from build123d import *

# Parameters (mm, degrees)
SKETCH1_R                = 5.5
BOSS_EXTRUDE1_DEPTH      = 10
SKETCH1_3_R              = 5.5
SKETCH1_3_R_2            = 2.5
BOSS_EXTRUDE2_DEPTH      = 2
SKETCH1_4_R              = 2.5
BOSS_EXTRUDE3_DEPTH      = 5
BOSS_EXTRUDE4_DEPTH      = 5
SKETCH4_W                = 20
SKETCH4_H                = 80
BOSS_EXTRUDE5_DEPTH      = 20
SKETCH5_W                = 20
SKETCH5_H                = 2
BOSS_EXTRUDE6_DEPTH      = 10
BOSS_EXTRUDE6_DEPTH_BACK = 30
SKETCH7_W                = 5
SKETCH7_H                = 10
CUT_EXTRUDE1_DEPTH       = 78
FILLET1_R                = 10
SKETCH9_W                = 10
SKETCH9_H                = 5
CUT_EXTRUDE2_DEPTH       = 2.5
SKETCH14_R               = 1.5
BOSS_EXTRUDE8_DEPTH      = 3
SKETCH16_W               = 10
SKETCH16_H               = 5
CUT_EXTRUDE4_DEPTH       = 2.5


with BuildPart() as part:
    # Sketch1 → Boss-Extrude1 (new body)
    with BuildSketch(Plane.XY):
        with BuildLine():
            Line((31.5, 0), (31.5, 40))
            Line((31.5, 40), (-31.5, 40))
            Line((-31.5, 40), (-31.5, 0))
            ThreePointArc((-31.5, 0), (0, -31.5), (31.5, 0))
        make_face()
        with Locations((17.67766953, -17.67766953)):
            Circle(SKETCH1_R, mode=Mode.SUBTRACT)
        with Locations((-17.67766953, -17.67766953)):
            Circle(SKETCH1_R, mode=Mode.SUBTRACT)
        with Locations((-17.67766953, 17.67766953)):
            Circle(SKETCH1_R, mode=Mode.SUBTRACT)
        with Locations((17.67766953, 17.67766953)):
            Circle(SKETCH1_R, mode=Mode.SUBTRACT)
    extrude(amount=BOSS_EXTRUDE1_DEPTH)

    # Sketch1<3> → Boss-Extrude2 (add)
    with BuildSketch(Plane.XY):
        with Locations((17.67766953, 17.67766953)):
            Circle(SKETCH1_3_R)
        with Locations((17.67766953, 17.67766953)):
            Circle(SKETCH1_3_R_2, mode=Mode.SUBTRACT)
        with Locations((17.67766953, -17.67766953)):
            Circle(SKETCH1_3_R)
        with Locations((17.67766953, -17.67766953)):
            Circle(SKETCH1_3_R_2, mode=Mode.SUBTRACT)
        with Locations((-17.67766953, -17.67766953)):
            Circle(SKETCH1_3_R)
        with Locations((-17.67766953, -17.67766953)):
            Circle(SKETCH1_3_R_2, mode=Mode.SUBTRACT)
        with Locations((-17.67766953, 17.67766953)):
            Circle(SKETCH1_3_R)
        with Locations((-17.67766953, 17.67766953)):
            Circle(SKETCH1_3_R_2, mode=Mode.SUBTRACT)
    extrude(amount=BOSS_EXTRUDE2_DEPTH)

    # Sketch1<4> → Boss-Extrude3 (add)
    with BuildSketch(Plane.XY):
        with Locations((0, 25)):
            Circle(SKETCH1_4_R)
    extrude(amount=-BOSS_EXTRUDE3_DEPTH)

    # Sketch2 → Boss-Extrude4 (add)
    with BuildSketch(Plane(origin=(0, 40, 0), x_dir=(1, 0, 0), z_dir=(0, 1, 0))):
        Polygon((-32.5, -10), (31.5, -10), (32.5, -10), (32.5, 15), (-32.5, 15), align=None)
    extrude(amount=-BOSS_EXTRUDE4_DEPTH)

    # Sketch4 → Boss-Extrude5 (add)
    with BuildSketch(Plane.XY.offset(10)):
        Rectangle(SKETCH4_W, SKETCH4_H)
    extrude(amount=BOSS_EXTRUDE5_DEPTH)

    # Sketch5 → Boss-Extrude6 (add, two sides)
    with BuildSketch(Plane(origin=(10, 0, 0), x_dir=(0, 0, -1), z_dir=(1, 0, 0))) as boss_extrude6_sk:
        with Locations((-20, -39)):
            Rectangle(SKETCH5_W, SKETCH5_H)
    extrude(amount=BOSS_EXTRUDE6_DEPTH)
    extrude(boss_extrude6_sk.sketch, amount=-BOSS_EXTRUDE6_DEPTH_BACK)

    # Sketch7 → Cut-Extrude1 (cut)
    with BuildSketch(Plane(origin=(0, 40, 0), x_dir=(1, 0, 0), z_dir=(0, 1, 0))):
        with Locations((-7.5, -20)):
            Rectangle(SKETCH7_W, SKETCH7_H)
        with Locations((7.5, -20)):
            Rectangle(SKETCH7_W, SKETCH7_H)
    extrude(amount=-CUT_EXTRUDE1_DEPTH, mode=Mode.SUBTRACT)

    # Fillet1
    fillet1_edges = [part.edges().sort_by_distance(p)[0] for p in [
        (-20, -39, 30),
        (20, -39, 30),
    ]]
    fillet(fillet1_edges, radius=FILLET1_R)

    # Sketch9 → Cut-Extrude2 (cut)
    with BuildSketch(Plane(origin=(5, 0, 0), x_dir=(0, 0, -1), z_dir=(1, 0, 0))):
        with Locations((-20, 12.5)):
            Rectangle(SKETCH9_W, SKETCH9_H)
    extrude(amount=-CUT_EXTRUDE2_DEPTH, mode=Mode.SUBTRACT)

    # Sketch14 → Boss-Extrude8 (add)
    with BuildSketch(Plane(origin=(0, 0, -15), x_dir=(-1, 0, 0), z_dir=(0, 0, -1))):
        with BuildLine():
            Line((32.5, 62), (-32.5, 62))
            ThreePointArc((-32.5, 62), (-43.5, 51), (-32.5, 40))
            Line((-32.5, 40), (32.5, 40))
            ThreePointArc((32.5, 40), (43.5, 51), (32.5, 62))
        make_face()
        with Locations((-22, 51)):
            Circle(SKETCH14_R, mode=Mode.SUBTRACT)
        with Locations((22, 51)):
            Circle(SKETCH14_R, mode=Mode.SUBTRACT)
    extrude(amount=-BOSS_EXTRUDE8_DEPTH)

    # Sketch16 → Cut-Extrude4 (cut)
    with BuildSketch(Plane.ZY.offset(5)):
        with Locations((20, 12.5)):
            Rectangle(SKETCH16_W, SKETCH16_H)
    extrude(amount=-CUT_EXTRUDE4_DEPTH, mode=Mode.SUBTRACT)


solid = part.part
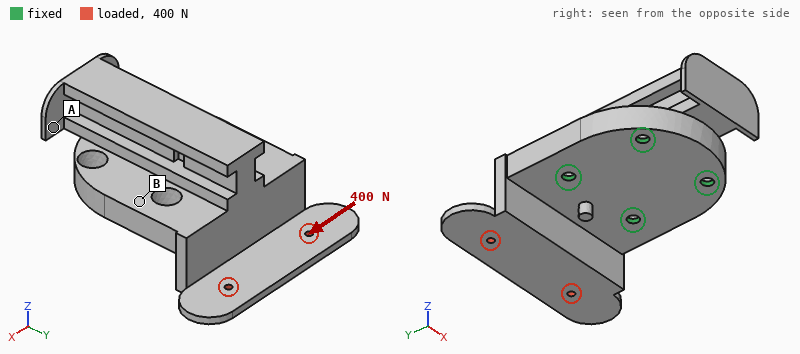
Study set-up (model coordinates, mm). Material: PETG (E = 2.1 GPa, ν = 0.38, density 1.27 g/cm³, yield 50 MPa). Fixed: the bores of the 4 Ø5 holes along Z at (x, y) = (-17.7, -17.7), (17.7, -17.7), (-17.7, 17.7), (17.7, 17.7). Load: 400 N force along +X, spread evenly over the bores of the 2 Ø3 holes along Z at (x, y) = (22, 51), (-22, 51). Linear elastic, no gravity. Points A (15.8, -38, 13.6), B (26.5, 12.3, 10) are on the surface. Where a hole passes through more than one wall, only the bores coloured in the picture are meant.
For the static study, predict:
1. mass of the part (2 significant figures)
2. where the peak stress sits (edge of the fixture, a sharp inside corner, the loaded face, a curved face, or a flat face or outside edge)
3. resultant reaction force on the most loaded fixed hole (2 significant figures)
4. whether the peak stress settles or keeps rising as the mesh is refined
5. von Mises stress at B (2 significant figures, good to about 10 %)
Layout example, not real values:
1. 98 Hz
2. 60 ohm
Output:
1. 92 g
2. edge of the fixture
3. 340 N
4. keeps rising
5. 3.2 MPa
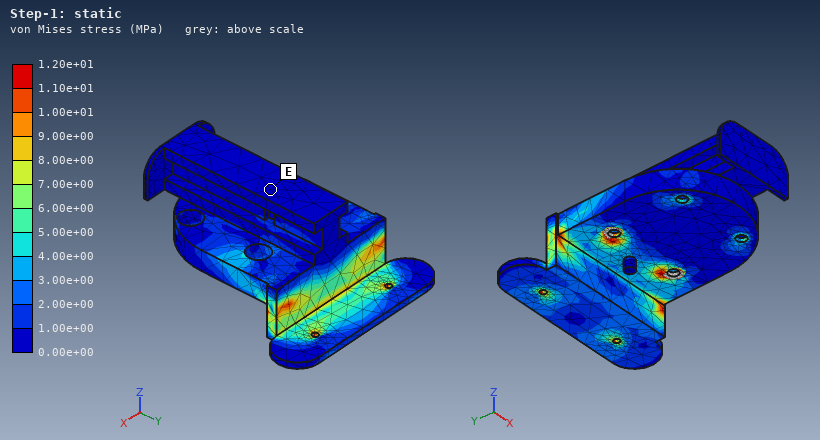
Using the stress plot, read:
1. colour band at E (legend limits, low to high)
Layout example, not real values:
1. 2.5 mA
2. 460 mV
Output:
1. 0.00e+00 to 1.00e+00 MPa
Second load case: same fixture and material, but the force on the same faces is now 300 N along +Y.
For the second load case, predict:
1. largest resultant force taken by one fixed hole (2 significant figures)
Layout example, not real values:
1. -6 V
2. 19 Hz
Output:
1. 170 N
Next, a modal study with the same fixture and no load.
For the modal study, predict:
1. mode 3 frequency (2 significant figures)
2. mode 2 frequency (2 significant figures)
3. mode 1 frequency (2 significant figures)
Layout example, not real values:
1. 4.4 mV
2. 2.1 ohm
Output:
1. 1400 Hz
2. 840 Hz
3. 700 Hz
